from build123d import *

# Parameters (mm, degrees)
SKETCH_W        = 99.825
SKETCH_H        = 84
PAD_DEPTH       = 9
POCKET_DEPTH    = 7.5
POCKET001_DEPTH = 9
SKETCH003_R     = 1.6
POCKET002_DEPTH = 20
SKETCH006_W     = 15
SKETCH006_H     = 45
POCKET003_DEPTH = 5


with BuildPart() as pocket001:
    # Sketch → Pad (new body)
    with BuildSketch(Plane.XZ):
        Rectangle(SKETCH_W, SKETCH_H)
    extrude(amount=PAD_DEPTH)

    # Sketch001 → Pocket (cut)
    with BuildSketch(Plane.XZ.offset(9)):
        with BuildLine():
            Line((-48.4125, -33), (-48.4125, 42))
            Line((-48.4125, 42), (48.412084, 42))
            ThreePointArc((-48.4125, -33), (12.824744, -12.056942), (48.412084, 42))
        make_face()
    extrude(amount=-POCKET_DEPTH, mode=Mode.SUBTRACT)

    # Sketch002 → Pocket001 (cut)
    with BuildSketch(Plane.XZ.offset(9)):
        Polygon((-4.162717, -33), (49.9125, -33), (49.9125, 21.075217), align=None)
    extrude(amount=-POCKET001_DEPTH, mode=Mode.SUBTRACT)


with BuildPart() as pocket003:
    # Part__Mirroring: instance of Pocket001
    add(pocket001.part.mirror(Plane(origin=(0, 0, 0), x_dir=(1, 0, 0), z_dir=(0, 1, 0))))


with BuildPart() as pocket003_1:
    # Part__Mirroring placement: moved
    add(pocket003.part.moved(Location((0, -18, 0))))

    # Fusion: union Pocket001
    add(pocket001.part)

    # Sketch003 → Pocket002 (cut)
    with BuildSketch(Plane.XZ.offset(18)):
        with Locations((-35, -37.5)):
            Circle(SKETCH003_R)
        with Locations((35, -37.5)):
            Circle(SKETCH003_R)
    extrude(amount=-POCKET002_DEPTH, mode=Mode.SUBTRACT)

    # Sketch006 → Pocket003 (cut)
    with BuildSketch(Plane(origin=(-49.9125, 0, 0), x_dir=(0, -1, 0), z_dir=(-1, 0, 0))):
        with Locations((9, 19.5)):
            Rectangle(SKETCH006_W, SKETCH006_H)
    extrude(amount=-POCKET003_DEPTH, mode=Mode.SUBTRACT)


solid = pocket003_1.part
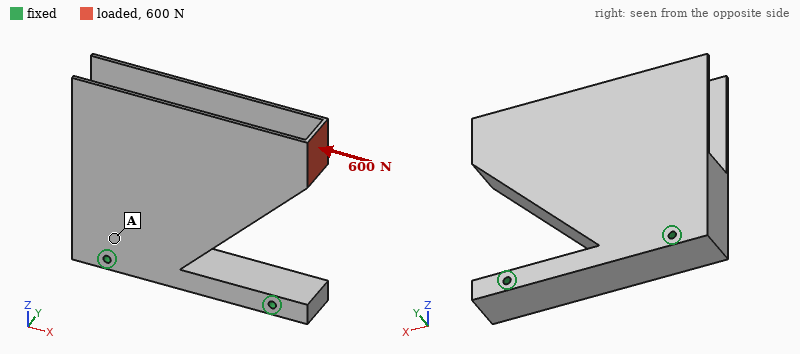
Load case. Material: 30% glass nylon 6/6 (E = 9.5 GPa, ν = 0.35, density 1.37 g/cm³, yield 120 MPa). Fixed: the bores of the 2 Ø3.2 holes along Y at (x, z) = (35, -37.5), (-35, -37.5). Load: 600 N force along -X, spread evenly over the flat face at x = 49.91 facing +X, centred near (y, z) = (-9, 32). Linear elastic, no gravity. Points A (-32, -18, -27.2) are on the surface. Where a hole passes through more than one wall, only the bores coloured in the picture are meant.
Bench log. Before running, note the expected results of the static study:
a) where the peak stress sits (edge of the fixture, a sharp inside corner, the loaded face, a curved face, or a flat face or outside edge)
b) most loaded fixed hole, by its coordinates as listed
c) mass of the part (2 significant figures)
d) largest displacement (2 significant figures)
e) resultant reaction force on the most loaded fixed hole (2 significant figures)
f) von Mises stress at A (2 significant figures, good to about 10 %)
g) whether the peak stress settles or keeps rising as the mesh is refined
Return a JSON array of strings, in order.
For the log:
["edge of the fixture", "(-35, -37.5)", "58 g", "1.4 mm", "620 N", "12 MPa", "keeps rising"]
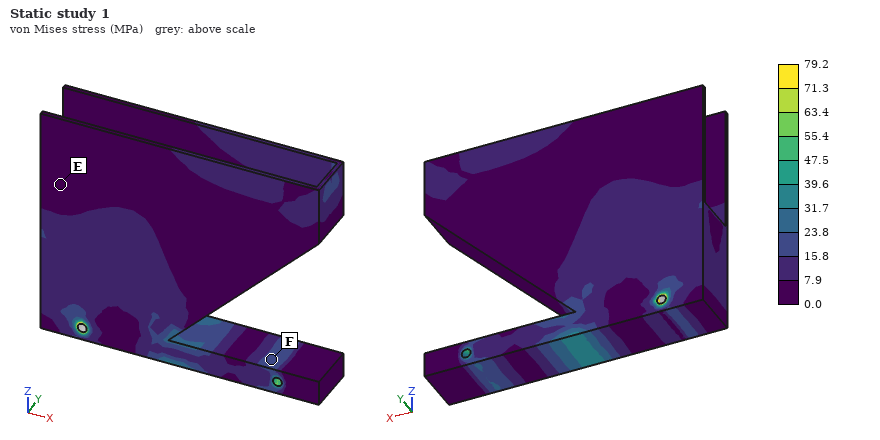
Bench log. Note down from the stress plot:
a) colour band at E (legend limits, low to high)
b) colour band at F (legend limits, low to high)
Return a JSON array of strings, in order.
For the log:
["0.0 to 7.9 MPa", "15.8 to 23.8 MPa"]
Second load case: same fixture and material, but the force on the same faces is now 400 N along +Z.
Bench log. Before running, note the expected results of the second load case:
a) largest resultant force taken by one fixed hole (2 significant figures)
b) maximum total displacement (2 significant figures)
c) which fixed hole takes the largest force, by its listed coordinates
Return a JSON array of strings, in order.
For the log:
["400 N", "1.1 mm", "(35, -37.5)"]
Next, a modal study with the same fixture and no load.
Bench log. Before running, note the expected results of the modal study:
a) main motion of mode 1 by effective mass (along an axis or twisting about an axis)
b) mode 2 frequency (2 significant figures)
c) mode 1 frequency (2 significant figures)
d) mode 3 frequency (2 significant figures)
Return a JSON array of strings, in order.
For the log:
["along Y", "290 Hz", "270 Hz", "510 Hz"]
